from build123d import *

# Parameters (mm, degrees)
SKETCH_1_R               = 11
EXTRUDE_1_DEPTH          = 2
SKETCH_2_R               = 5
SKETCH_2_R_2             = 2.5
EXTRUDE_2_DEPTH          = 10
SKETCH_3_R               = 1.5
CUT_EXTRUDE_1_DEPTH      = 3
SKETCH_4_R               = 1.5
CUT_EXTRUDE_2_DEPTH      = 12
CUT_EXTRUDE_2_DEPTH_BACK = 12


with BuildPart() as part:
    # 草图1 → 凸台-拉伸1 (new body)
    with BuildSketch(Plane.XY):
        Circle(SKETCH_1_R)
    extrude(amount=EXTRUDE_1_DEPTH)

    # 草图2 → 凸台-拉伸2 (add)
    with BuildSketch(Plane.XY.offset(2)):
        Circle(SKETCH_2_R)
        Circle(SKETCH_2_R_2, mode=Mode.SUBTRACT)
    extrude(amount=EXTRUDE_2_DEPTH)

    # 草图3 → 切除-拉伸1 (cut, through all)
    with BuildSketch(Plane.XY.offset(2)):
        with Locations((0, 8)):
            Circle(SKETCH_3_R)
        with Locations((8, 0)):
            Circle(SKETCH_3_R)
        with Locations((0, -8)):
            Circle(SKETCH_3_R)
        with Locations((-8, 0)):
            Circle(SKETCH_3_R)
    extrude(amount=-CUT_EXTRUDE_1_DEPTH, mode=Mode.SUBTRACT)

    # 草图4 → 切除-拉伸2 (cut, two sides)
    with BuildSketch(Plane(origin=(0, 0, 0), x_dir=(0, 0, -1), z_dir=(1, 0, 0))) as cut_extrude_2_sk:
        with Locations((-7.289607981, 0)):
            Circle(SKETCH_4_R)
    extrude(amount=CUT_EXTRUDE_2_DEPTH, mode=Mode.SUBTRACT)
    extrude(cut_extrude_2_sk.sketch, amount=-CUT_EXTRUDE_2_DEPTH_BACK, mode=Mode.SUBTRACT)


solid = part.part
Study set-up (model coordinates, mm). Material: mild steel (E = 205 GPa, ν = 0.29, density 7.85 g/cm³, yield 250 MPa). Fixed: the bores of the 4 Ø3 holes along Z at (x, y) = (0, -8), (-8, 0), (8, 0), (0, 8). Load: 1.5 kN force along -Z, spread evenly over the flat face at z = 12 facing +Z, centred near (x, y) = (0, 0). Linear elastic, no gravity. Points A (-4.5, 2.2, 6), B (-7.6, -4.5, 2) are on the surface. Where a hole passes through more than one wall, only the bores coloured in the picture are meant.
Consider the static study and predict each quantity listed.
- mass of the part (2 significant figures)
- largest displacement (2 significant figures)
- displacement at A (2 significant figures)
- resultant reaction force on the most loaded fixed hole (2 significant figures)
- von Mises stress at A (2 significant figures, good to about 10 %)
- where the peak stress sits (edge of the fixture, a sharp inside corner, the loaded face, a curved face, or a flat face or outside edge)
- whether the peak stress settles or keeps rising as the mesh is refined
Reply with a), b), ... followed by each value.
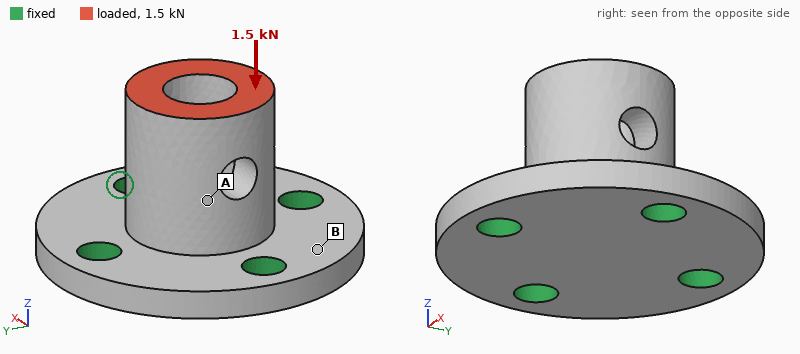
a) 9.9 g
b) 4.0 µm
c) 2.8 µm
d) 400 N
e) 42 MPa
f) edge of the fixture
g) keeps rising
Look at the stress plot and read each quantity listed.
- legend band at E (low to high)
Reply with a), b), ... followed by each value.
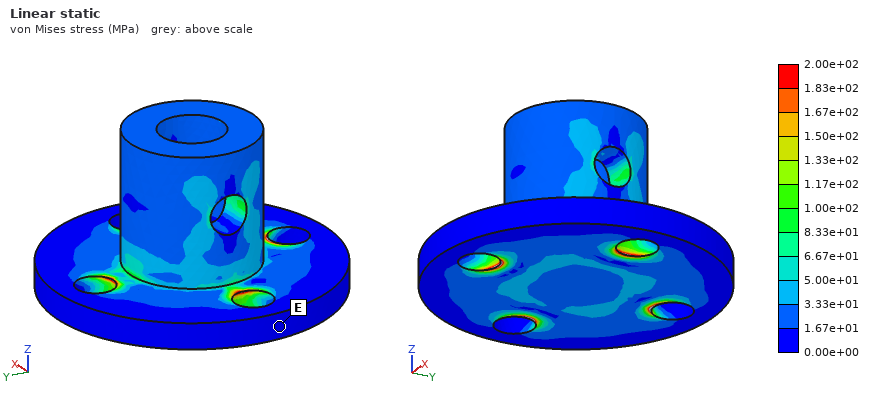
a) 0.00e+00 to 1.67e+01 MPa
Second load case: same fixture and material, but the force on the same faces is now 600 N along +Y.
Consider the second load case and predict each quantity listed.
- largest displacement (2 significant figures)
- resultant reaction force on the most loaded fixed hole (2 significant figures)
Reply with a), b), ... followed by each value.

a) 12 µm
b) 540 N
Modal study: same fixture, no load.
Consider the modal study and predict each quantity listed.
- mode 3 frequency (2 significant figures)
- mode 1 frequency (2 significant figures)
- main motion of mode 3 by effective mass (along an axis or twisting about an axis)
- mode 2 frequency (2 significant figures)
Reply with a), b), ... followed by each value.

a) 50 kHz
b) 29 kHz
c) along Z
d) 30 kHz
